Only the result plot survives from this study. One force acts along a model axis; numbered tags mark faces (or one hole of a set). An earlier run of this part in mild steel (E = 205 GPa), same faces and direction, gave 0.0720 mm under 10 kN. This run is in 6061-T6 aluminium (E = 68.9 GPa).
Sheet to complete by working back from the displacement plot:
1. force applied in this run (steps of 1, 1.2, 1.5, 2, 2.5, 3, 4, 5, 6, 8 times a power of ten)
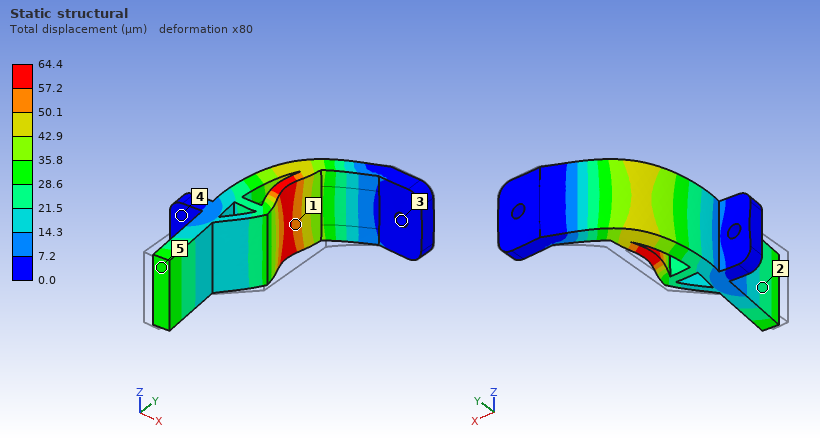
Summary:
3 kN
